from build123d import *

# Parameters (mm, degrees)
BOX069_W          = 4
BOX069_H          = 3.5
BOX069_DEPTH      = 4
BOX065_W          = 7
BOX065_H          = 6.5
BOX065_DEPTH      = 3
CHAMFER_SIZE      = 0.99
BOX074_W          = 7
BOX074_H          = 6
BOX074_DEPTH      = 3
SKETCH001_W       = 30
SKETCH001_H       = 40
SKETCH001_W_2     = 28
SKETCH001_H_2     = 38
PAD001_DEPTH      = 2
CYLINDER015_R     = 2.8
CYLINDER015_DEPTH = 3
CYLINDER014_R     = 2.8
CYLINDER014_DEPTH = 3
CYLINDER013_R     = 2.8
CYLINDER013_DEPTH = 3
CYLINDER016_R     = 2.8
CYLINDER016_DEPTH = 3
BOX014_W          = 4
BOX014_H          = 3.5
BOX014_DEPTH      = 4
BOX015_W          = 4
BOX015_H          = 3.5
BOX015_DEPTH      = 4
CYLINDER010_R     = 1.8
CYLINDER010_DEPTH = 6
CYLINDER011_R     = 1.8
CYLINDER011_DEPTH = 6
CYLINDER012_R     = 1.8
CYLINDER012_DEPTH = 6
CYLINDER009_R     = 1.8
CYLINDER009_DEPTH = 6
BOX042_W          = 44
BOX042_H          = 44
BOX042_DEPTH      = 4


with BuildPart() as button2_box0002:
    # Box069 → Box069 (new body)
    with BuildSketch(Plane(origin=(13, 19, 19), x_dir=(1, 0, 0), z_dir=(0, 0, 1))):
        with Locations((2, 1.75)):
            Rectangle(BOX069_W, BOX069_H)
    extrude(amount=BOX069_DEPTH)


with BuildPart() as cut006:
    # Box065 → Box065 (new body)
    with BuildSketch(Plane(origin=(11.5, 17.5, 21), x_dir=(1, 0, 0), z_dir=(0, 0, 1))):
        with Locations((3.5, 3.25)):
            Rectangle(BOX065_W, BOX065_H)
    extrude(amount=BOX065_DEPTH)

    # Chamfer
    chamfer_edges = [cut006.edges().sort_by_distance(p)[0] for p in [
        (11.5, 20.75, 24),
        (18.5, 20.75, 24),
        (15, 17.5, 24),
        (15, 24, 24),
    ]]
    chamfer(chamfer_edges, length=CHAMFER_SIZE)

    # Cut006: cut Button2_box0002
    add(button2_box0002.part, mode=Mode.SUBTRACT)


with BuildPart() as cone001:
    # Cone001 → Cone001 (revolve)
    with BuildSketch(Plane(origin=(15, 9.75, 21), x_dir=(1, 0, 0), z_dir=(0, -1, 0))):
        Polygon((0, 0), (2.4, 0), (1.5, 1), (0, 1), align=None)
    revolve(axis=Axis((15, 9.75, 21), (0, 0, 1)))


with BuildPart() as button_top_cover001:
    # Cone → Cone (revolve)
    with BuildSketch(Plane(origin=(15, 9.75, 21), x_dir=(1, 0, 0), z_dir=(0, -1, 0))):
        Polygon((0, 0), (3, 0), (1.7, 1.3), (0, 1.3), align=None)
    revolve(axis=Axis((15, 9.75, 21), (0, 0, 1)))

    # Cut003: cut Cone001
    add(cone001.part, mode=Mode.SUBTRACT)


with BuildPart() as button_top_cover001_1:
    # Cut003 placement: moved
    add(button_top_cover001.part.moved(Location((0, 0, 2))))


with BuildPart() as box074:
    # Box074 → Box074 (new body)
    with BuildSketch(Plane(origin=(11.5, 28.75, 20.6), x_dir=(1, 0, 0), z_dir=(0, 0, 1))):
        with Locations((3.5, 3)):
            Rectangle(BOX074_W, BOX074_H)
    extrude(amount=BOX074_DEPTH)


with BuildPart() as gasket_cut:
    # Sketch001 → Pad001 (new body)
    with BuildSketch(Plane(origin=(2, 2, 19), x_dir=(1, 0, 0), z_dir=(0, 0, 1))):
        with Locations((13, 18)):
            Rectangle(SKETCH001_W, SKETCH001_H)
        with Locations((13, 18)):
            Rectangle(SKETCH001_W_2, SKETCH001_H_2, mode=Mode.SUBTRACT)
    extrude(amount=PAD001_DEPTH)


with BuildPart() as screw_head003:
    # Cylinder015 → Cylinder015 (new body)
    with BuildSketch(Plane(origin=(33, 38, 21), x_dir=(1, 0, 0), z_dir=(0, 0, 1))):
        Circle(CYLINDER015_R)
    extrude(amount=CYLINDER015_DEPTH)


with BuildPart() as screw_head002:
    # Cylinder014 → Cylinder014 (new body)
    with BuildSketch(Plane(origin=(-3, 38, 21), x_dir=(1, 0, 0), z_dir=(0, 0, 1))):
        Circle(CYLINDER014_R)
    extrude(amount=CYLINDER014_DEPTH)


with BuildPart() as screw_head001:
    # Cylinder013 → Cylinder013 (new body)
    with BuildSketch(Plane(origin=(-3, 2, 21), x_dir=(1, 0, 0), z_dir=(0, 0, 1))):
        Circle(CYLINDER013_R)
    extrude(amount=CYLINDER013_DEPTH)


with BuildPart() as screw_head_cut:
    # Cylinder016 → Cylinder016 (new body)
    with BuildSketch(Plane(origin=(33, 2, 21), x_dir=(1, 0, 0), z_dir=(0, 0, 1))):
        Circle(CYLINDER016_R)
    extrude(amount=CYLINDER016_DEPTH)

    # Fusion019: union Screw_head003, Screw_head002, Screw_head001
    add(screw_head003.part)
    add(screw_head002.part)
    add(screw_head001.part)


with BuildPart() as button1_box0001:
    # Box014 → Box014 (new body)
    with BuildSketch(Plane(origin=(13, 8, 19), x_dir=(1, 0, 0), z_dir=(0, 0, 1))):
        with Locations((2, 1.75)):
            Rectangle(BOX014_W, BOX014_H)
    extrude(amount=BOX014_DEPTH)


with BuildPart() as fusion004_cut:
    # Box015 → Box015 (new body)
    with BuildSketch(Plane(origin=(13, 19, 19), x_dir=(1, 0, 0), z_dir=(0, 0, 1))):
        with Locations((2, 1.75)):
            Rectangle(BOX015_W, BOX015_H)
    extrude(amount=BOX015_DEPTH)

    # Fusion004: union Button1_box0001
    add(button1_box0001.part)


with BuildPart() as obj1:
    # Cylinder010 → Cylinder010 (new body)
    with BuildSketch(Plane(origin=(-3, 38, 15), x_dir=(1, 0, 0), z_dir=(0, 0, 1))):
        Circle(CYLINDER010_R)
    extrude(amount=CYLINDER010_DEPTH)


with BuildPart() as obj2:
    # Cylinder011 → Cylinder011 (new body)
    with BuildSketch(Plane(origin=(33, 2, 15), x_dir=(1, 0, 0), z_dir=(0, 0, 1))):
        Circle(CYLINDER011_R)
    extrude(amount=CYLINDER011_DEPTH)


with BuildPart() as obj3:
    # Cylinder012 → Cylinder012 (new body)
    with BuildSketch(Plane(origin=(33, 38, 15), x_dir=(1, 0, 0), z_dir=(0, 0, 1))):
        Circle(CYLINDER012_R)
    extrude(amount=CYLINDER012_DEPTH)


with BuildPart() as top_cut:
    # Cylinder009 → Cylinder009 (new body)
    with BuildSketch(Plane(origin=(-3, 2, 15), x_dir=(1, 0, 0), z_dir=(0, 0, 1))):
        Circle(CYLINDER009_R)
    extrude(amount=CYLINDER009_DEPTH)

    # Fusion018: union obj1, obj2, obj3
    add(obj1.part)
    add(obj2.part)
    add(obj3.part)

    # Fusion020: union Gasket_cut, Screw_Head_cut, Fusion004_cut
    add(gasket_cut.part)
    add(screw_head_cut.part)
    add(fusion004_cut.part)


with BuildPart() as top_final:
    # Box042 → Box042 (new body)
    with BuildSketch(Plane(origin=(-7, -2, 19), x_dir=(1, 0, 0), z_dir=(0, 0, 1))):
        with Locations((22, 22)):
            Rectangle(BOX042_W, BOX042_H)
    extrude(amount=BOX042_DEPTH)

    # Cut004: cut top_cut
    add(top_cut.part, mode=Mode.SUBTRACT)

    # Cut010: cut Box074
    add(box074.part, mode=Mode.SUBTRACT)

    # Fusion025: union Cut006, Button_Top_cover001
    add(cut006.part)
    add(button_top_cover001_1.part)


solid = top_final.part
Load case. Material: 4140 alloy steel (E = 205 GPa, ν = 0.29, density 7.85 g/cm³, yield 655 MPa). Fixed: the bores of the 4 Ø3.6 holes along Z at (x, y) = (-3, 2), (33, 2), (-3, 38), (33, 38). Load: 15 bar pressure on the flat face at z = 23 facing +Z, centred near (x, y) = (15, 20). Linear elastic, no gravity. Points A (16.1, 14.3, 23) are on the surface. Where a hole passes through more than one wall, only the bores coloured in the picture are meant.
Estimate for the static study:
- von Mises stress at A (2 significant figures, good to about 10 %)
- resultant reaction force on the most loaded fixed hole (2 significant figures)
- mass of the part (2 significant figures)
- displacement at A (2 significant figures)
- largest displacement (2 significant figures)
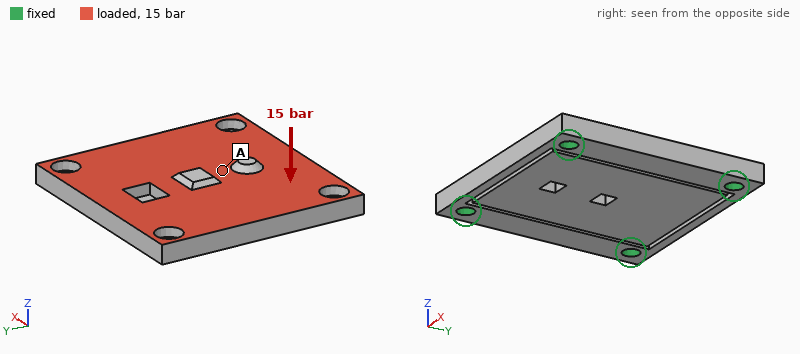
46 MPa
780 N
55 g
22 µm
23 µm
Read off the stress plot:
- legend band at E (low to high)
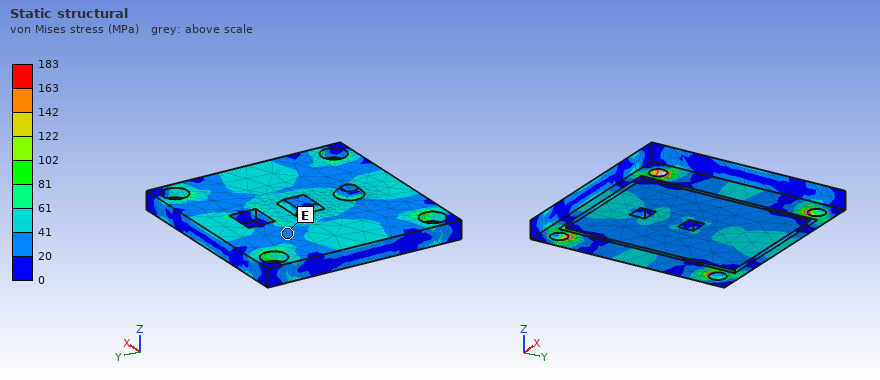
20 to 41 MPa
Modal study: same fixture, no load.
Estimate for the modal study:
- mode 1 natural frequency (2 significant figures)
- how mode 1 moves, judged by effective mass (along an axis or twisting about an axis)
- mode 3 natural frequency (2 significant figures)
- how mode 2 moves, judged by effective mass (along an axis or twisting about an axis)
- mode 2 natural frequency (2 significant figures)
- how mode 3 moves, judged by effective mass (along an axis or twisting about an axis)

8400 Hz
along Z
14 kHz
twisting about X
13 kHz
twisting about Y
